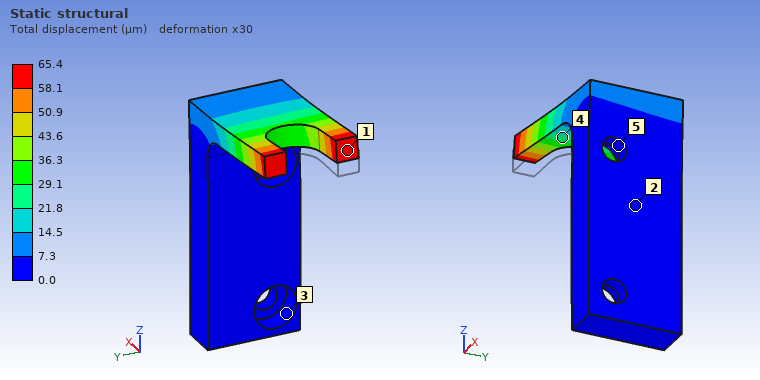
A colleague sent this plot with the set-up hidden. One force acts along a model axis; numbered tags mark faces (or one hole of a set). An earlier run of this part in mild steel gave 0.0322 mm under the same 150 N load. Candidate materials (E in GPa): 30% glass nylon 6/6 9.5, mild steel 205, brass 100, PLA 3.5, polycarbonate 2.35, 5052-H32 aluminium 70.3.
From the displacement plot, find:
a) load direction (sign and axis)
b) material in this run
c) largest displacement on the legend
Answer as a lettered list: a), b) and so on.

a) +Z
b) brass
c) 65.4 µm
